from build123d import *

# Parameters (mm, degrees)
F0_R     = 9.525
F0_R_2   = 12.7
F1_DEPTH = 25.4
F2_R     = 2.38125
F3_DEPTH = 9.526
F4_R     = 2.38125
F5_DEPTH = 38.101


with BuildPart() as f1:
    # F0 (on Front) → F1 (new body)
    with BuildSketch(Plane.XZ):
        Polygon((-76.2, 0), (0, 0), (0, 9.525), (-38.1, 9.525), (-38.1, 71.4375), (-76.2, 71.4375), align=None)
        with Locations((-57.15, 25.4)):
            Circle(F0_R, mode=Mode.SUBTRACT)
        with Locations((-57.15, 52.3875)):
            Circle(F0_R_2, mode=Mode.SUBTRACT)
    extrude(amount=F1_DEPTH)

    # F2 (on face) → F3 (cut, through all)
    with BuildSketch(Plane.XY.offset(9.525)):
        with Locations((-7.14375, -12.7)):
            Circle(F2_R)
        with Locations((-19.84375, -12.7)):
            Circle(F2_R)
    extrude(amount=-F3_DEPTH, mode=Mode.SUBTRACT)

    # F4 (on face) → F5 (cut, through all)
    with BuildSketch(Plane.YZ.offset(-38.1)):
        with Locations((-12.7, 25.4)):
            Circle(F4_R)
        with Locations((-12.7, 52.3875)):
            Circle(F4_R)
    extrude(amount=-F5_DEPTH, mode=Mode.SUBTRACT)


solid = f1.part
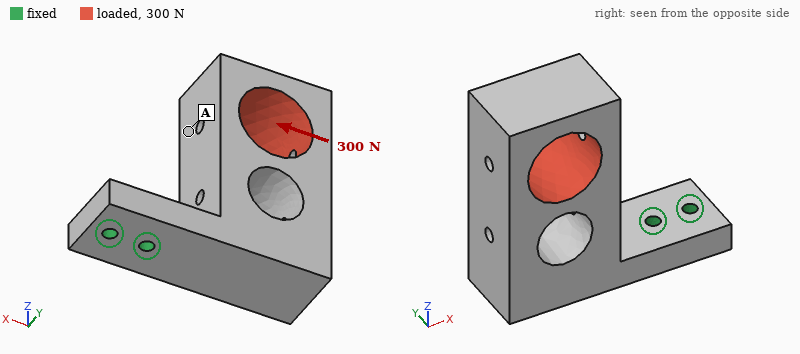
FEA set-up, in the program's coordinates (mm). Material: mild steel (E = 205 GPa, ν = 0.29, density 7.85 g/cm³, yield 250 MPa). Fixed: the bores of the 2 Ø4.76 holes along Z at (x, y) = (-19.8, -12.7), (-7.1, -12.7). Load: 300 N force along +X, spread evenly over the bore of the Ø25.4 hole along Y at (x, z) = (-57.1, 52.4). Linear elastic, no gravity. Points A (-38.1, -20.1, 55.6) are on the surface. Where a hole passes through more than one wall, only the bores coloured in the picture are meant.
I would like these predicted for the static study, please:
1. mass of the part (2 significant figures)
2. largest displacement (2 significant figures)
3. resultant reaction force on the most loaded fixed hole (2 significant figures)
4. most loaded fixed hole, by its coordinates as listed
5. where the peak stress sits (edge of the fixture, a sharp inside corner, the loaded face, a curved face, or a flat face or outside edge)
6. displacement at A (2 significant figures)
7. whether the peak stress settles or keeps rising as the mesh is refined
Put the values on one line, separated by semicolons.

450 g; 76 µm; 430 N; (-19.8, -12.7); edge of the fixture; 49 µm; keeps rising
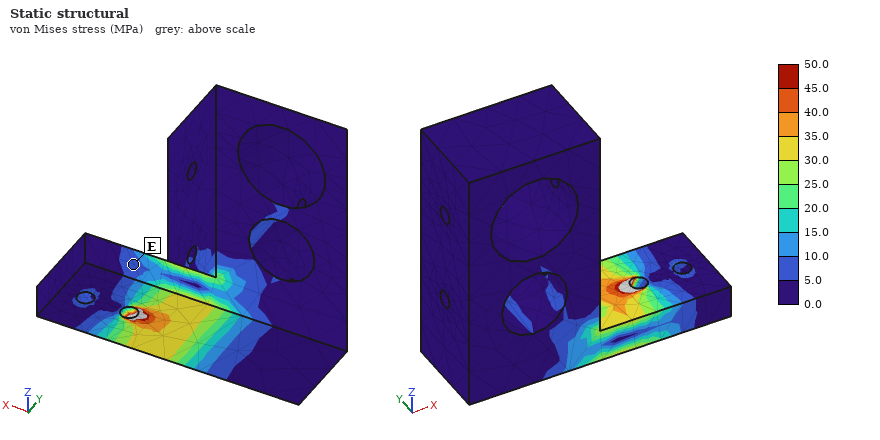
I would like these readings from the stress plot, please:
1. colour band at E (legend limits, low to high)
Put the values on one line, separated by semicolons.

5.0 to 10.0 MPa
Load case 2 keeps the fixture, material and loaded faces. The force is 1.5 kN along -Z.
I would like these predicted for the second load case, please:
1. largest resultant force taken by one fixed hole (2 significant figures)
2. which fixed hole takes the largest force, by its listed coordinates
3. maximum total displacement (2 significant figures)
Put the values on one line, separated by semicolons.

2.8 kN; (-19.8, -12.7); 0.21 mm
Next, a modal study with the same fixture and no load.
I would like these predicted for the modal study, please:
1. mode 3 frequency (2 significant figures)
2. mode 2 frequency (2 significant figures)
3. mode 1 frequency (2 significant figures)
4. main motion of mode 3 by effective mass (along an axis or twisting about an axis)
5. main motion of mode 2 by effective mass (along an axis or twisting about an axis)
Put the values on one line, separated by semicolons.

2800 Hz; 970 Hz; 690 Hz; along Y; along Y
